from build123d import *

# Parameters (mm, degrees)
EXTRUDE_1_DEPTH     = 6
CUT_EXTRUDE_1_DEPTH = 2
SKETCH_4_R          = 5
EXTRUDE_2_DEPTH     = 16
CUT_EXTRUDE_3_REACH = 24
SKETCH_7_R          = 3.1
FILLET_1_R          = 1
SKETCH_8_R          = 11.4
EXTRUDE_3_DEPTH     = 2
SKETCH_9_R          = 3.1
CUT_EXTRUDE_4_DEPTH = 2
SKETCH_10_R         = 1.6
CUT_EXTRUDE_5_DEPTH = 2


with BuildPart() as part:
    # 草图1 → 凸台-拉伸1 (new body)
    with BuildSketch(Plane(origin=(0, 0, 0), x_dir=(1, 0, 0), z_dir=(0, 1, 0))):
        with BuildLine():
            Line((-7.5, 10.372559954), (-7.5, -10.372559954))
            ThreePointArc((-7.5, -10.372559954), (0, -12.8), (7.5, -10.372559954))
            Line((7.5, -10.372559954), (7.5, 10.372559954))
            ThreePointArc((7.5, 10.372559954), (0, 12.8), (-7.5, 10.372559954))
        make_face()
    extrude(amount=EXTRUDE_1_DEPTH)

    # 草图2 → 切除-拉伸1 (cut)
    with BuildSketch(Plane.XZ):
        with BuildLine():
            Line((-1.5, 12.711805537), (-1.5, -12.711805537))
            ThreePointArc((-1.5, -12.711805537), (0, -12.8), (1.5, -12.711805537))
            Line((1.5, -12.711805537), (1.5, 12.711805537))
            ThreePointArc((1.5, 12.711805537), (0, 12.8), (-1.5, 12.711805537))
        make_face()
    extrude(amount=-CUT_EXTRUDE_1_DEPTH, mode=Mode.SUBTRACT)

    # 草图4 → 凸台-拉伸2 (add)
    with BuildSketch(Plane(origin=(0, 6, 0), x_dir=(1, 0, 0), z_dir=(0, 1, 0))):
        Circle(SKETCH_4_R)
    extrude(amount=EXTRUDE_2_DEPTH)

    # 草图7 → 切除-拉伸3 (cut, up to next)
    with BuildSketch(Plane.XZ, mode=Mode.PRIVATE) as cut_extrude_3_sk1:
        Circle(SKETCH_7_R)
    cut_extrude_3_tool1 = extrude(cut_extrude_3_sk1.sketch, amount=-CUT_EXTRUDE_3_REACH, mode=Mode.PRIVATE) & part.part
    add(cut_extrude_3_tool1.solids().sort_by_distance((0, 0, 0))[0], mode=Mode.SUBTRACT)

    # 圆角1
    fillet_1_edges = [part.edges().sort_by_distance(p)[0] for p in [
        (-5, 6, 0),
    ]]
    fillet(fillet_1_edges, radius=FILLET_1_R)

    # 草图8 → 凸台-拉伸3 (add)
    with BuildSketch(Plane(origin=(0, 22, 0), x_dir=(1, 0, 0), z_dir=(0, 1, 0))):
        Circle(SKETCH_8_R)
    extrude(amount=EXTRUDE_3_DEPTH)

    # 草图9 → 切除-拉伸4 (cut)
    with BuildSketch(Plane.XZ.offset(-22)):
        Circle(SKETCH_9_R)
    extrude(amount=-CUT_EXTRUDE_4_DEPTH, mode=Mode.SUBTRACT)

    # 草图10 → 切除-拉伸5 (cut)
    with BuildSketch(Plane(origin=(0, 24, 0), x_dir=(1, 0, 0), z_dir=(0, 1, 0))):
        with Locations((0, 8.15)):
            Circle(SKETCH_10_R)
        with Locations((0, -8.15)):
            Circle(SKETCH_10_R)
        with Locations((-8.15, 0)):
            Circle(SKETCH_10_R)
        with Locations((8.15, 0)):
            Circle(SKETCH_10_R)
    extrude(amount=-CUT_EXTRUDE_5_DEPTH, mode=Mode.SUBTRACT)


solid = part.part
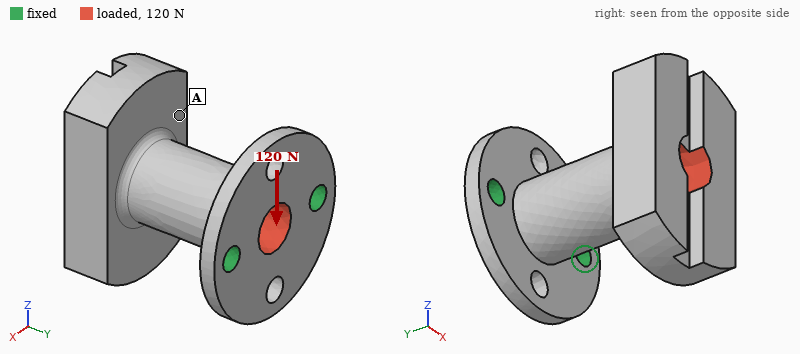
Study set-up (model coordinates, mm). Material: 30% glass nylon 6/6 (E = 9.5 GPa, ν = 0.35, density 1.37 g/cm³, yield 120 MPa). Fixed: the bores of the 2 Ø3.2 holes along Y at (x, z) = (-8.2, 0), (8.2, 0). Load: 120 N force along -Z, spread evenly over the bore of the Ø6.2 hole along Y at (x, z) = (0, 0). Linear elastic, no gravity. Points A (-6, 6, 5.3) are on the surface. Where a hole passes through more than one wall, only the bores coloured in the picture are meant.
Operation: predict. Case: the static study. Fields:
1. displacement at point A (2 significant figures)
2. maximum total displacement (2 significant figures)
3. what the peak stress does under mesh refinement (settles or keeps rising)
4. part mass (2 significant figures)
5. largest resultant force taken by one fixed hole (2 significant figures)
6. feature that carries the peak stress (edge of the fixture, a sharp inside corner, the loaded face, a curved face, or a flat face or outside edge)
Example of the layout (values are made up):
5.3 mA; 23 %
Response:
0.31 mm; 0.46 mm; keeps rising; 4.6 g; 60 N; edge of the fixture
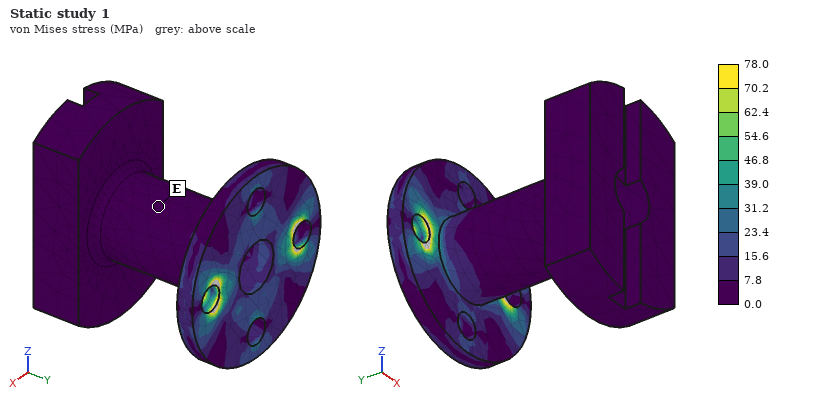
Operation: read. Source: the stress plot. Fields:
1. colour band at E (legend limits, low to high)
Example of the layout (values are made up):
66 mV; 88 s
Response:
0.0 to 7.8 MPa
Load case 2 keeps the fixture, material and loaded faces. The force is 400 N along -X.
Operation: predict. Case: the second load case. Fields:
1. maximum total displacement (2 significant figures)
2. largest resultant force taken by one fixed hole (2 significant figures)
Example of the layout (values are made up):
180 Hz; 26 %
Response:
0.35 mm; 410 N
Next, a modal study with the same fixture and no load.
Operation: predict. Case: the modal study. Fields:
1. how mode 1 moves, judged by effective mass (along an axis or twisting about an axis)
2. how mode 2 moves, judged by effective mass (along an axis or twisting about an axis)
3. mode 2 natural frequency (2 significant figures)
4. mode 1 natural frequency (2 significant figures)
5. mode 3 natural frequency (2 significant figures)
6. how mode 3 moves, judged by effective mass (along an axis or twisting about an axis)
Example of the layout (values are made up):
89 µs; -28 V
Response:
along Z; along X; 2400 Hz; 1200 Hz; 4500 Hz; twisting about Y
